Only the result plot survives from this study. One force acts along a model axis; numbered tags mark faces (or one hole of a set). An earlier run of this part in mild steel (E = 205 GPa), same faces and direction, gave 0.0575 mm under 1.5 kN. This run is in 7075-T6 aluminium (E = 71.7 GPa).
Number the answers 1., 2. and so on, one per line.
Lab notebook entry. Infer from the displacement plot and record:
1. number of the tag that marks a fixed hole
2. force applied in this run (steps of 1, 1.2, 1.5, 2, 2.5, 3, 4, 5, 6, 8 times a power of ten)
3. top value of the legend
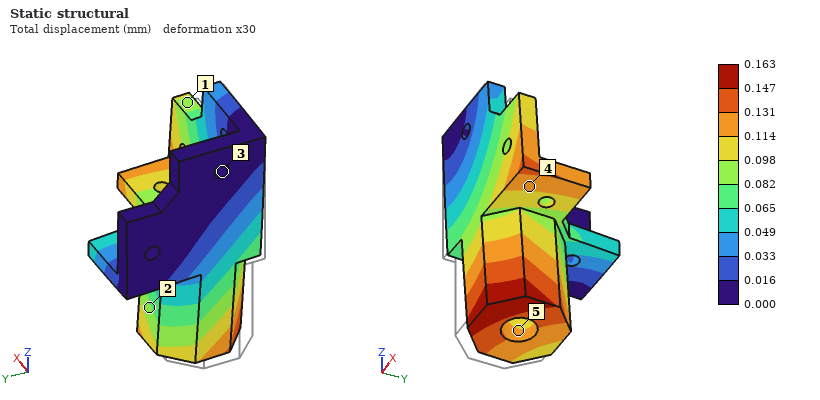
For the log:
1. 3
2. 1.5 kN
3. 0.163 mm
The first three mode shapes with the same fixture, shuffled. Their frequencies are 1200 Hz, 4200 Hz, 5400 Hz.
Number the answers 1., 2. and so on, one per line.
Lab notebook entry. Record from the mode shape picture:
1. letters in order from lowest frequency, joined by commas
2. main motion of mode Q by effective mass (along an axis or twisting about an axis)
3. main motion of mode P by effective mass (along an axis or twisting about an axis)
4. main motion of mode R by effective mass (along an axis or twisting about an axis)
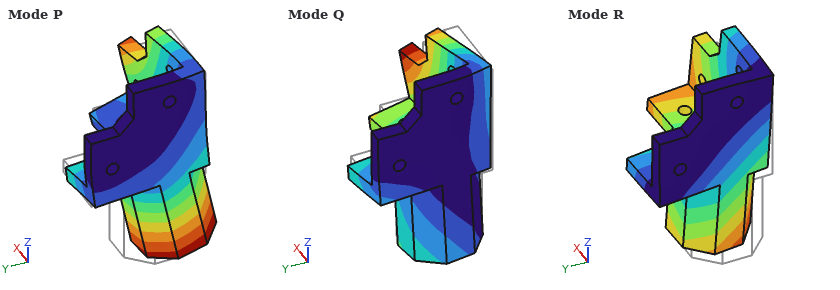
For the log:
1. R, Q, P
2. along Y
3. along Y
4. along X
